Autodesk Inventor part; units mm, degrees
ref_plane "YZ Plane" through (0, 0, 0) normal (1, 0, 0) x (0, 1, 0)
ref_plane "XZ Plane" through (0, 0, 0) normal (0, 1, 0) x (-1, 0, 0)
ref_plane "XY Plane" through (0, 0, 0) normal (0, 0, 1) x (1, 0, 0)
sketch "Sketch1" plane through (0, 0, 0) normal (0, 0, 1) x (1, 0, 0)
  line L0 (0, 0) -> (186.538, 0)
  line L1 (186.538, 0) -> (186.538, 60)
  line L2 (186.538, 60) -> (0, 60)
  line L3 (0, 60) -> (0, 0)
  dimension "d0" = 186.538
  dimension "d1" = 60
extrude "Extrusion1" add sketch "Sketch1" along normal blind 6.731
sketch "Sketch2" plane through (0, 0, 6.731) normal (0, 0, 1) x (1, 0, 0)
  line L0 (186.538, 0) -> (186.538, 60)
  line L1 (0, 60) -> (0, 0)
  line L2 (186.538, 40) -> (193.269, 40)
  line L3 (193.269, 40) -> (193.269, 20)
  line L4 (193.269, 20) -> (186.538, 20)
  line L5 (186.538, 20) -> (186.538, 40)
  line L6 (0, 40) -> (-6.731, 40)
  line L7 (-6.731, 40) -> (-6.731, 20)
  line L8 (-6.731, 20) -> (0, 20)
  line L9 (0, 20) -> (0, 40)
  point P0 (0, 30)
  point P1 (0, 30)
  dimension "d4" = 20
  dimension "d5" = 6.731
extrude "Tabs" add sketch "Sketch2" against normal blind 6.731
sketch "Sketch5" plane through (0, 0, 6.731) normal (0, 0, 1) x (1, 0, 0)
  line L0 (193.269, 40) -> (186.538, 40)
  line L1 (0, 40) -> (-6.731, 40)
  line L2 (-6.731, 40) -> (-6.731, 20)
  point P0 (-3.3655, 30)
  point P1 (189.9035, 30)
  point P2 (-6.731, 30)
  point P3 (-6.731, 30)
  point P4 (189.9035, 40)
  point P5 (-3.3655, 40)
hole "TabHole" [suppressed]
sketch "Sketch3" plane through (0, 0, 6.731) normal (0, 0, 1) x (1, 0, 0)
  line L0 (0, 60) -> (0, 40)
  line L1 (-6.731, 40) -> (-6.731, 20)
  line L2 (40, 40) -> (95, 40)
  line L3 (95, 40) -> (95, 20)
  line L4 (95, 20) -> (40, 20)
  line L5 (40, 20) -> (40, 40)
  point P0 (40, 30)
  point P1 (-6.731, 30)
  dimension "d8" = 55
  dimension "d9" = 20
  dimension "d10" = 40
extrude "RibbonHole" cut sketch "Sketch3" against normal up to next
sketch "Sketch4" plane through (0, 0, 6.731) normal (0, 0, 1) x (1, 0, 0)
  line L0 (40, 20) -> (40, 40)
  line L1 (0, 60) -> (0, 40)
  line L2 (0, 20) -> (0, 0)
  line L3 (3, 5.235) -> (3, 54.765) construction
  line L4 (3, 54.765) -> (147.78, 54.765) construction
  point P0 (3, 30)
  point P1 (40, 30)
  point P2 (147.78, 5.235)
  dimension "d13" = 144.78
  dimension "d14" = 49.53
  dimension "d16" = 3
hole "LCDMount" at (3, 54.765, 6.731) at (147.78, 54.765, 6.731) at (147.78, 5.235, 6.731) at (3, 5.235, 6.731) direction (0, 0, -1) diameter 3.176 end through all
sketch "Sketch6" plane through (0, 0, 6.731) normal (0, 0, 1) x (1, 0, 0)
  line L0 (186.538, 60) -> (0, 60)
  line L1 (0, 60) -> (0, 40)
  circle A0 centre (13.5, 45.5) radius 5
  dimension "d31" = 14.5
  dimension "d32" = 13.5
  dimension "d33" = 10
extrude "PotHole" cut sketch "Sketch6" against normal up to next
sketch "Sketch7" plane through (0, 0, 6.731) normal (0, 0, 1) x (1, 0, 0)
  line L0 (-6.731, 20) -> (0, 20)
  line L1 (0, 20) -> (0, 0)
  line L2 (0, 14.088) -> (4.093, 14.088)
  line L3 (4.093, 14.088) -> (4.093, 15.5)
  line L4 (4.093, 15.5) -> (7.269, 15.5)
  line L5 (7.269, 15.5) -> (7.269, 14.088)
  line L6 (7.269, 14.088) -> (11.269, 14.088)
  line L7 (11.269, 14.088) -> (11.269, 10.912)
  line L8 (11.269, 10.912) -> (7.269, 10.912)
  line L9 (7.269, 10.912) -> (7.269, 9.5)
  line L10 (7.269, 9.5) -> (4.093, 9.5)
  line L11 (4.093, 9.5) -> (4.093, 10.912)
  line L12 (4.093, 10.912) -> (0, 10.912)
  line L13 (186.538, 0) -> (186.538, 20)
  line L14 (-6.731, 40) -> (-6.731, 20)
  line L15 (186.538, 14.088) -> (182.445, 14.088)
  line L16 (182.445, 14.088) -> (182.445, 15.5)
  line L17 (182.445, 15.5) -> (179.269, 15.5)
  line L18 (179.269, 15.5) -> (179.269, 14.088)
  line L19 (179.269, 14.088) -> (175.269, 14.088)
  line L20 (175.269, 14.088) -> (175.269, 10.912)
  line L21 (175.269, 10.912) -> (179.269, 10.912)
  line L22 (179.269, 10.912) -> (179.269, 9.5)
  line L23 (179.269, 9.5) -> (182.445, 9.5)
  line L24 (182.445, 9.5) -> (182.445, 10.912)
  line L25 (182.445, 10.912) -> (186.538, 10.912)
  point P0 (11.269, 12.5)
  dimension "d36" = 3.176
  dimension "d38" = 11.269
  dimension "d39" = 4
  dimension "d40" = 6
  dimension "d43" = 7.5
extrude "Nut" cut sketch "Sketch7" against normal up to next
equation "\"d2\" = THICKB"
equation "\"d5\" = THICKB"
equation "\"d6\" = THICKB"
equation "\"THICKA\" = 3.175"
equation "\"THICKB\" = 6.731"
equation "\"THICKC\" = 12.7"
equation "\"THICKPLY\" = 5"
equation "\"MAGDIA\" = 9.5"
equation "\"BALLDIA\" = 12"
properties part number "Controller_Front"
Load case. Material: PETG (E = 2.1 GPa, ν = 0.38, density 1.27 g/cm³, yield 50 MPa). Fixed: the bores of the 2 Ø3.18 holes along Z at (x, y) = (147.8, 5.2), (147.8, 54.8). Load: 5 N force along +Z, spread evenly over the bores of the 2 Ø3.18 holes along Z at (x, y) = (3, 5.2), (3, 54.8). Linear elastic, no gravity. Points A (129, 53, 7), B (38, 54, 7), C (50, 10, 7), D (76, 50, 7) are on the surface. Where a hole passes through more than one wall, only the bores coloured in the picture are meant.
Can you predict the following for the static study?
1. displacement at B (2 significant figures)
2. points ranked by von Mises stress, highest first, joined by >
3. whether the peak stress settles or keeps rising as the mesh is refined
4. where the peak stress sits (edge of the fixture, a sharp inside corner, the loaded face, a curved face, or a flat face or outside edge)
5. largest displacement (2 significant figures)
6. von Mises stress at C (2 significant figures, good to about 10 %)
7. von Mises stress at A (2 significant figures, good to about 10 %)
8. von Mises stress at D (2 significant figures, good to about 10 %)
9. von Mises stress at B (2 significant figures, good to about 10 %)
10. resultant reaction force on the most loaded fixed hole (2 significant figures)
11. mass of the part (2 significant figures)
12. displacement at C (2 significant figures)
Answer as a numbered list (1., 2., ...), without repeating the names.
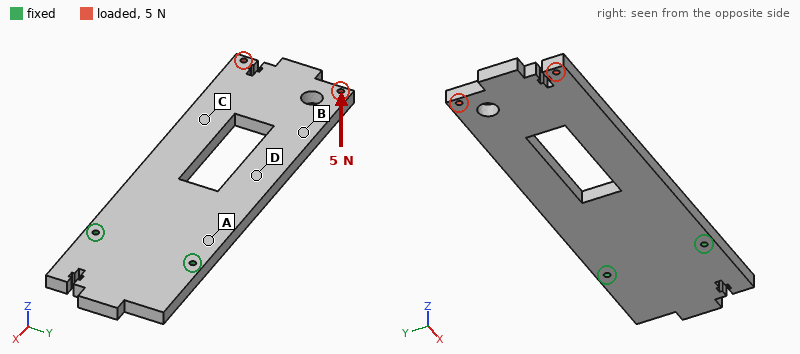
1. 1.3 mm
2. A > D > C > B
3. keeps rising
4. edge of the fixture
5. 2.2 mm
6. 0.79 MPa
7. 1.5 MPa
8. 1.2 MPa
9. 0.53 MPa
10. 2.5 N
11. 87 g
12. 1.0 mm
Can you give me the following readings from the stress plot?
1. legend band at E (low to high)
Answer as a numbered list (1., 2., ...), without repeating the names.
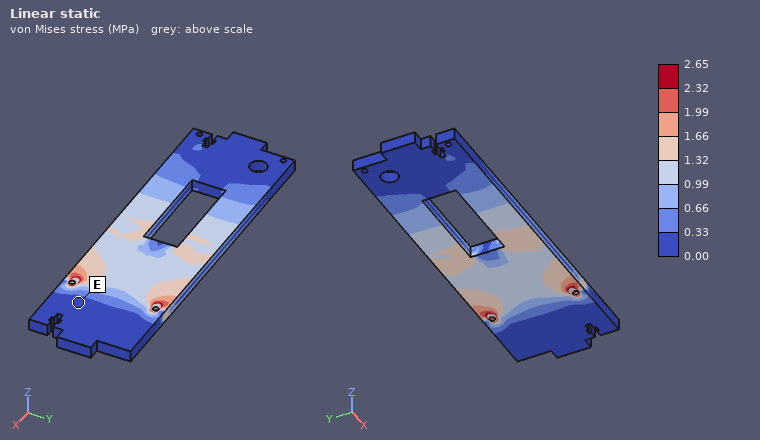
1. 0.00 to 0.33 MPa
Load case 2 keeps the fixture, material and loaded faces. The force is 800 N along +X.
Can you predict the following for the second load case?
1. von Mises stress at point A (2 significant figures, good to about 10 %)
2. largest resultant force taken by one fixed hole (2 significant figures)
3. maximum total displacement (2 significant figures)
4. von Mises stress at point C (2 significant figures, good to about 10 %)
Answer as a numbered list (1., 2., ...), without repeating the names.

1. 2.5 MPa
2. 400 N
3. 0.26 mm
4. 3.0 MPa
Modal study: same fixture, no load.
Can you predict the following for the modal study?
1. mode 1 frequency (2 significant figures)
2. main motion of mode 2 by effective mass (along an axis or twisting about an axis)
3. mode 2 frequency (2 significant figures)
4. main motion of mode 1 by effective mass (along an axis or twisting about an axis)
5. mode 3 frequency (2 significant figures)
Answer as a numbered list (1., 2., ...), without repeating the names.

1. 59 Hz
2. twisting about X
3. 280 Hz
4. along Z
5. 350 Hz
